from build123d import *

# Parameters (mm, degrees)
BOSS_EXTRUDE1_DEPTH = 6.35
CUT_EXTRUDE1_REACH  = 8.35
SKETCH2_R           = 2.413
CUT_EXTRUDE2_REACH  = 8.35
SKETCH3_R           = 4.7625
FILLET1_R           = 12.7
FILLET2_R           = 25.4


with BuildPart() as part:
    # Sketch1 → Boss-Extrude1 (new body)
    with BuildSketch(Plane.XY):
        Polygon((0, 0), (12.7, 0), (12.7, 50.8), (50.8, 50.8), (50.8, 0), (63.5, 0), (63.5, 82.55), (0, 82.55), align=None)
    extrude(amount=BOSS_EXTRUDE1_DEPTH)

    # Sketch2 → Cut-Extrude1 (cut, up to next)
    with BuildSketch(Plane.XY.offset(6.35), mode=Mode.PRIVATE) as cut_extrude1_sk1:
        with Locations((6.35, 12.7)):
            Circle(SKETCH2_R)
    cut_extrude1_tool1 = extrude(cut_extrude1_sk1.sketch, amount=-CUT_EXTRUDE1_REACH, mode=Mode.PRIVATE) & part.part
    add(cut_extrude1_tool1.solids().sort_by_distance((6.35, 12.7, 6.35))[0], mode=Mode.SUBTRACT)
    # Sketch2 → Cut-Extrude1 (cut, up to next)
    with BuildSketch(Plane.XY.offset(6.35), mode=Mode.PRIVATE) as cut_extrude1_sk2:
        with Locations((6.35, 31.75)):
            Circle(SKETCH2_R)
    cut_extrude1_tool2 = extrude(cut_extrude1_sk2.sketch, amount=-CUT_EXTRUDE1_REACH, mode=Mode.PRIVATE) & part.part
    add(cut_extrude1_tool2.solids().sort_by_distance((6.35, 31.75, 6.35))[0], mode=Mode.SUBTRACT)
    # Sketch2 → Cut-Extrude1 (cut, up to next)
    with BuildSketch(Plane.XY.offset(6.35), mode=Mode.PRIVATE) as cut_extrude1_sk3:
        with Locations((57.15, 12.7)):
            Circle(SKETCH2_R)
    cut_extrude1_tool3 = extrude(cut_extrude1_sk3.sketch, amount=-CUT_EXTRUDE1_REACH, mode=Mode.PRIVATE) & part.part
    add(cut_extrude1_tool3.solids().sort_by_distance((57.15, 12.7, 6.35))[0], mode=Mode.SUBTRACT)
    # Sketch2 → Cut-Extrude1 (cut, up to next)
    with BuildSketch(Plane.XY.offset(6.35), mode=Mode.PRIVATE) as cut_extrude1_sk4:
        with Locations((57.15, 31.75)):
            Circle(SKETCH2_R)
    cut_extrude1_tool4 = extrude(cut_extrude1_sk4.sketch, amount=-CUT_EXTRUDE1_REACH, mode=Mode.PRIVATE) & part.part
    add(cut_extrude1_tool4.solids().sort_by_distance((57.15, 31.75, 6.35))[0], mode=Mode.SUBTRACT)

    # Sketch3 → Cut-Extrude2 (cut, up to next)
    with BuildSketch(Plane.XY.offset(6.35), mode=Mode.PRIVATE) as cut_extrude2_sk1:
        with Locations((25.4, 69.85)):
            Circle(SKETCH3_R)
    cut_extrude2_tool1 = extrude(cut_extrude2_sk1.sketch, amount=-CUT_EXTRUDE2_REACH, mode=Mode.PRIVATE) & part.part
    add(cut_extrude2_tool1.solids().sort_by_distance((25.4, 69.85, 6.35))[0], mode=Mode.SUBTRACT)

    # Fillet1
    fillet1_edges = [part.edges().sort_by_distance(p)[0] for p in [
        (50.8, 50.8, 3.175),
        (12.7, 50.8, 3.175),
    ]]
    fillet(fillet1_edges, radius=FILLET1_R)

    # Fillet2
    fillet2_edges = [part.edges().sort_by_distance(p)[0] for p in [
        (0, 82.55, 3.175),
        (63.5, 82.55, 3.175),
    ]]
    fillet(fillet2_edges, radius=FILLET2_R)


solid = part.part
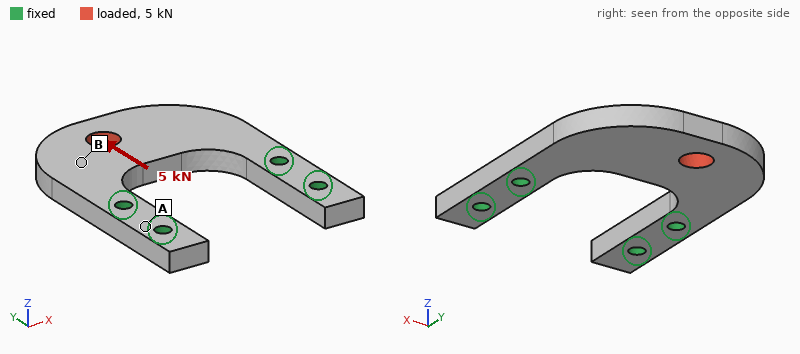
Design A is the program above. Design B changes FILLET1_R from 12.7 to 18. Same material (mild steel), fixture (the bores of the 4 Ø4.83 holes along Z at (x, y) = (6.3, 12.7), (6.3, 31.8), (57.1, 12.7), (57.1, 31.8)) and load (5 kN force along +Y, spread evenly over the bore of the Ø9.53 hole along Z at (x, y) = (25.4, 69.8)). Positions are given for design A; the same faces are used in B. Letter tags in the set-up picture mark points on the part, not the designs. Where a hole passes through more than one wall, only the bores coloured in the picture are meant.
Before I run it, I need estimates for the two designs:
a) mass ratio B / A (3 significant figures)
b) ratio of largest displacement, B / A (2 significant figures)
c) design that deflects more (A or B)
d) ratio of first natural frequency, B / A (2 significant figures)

1.02
0.91
A
1.0
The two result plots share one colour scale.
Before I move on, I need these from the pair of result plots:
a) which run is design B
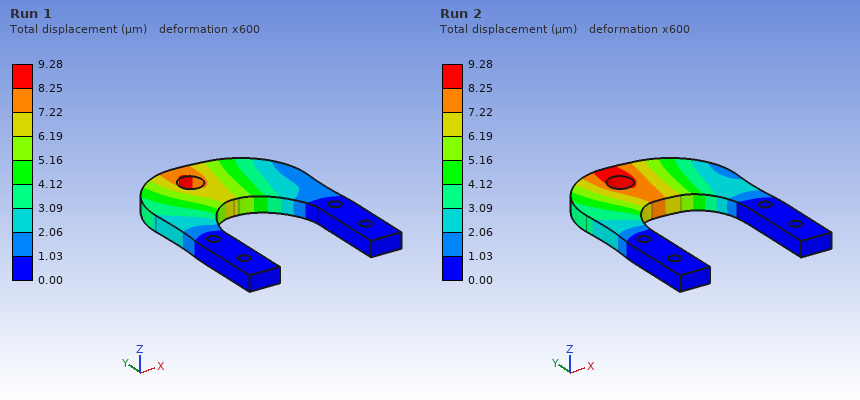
Run 1
